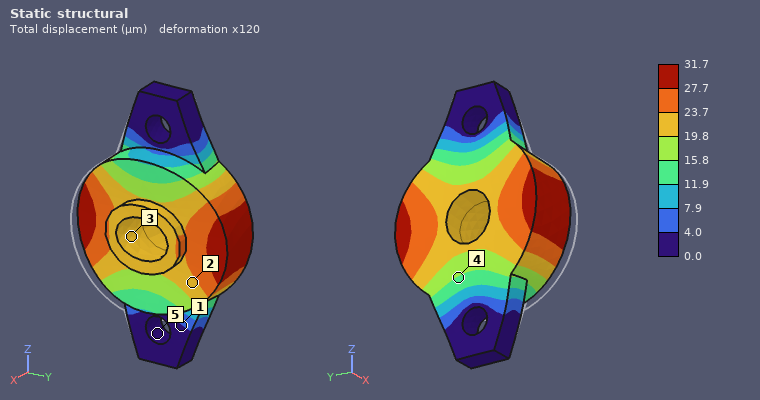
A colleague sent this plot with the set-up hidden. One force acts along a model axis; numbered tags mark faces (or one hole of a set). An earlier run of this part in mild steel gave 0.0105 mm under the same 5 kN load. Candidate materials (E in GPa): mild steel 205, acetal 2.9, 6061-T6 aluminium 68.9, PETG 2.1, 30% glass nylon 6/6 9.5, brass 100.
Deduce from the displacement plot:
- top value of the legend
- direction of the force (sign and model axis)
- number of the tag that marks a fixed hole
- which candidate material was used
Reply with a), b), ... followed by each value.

a) 31.7 µm
b) -X
c) 5
d) 6061-T6 aluminium
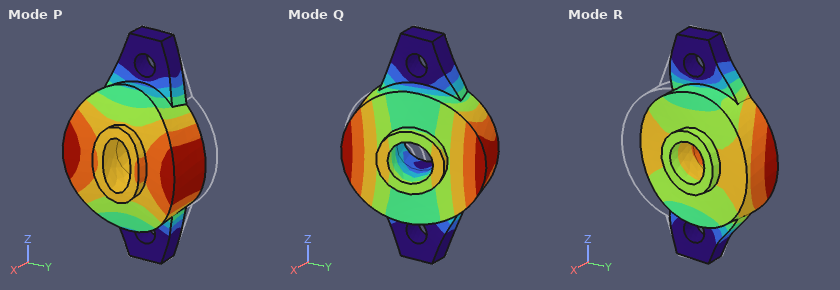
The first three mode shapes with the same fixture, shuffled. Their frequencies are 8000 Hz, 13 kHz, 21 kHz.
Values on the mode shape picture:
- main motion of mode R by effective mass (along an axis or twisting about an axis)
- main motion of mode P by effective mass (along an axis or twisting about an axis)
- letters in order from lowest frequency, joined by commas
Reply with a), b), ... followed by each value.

a) along Y
b) along X
c) Q, P, R
